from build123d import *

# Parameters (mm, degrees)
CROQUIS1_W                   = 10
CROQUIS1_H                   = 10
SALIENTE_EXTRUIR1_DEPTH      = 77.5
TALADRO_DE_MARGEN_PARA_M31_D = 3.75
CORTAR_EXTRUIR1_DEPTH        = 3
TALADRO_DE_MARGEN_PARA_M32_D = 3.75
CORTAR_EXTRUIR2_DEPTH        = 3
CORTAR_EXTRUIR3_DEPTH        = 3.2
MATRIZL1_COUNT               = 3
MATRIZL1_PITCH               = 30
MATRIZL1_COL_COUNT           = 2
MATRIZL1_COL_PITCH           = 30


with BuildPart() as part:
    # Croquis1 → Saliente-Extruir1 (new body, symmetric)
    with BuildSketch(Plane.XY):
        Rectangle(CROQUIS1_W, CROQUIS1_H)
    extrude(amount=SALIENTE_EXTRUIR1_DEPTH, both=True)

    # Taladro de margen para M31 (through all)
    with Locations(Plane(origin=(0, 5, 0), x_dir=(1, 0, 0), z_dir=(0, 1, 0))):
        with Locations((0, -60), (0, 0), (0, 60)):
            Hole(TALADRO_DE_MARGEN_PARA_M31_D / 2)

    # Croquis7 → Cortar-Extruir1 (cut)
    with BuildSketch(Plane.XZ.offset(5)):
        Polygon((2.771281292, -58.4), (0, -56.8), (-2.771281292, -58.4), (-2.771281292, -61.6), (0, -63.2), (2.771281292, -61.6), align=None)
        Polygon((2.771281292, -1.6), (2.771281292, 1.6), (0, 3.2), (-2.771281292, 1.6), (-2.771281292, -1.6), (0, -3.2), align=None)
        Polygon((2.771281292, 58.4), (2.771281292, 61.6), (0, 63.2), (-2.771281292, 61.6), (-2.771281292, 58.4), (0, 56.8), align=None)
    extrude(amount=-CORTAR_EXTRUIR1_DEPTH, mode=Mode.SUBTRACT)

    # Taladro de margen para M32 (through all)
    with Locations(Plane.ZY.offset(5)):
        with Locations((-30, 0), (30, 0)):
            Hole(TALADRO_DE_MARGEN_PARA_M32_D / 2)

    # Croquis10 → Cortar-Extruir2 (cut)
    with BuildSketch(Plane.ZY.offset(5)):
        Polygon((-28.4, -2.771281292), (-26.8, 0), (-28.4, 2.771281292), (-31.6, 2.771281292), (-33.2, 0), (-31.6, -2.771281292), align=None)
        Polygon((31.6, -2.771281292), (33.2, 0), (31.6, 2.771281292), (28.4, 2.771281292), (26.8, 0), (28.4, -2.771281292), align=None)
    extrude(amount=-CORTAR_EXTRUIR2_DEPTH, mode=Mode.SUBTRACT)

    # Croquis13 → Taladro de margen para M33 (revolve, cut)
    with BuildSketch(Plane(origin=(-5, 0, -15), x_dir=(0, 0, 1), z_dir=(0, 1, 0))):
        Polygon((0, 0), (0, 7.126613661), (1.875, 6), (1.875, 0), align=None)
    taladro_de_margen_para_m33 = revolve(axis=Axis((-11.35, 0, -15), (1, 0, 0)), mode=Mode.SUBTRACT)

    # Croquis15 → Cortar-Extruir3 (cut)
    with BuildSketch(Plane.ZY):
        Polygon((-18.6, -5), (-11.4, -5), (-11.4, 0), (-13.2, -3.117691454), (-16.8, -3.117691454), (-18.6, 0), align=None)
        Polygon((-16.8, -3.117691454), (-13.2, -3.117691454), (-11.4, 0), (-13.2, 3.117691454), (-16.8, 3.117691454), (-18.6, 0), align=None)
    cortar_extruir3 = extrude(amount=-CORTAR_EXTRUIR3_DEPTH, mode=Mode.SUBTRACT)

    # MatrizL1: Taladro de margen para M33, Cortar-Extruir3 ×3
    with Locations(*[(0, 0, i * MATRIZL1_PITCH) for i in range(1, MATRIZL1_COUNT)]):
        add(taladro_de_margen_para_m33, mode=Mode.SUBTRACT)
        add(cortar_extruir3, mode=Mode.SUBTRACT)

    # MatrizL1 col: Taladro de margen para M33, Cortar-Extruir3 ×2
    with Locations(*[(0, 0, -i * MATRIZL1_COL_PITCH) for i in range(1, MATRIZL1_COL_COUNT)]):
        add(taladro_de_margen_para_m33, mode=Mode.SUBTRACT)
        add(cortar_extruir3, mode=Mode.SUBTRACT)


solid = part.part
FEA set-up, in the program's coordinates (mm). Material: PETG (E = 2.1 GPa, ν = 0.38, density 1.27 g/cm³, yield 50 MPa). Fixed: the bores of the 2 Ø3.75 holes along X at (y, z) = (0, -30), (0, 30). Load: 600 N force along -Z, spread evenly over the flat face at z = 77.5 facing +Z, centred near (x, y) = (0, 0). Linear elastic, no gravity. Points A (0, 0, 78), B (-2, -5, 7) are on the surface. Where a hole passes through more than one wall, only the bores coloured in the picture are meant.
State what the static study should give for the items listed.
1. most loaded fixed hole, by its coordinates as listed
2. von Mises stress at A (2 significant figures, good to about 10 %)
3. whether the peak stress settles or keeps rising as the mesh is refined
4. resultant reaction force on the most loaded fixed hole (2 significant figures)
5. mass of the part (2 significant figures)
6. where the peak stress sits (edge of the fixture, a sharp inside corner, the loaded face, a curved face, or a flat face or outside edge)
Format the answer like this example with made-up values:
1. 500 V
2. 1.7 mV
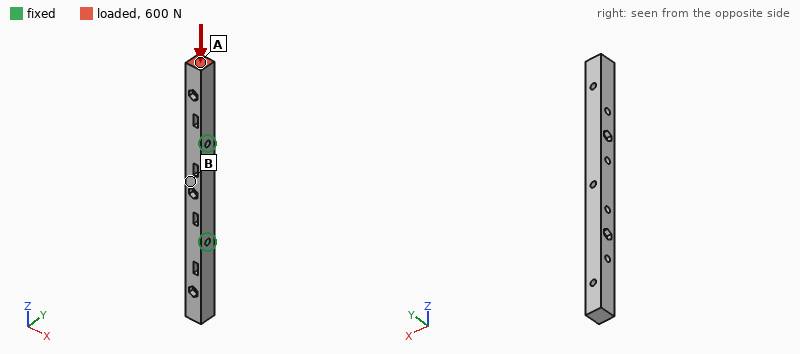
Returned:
1. (0, 30)
2. 6.0 MPa
3. keeps rising
4. 580 N
5. 18 g
6. edge of the fixture
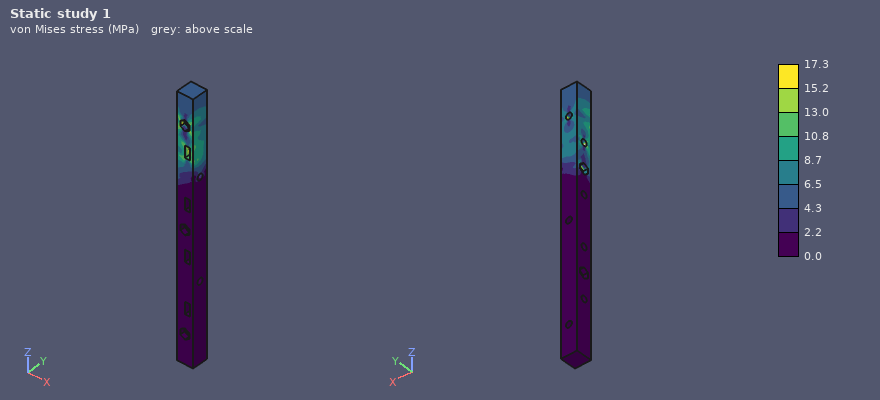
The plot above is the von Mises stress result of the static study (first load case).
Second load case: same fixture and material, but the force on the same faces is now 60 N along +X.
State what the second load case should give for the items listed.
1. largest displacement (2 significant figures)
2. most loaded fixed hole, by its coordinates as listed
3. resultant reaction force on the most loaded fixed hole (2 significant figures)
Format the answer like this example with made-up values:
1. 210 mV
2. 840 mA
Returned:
1. 1.7 mm
2. (0, 30)
3. 71 N
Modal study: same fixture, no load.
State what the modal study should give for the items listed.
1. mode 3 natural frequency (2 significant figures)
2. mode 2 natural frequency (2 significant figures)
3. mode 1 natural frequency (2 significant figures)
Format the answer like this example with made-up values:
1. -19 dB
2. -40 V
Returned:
1. 780 Hz
2. 760 Hz
3. 740 Hz
